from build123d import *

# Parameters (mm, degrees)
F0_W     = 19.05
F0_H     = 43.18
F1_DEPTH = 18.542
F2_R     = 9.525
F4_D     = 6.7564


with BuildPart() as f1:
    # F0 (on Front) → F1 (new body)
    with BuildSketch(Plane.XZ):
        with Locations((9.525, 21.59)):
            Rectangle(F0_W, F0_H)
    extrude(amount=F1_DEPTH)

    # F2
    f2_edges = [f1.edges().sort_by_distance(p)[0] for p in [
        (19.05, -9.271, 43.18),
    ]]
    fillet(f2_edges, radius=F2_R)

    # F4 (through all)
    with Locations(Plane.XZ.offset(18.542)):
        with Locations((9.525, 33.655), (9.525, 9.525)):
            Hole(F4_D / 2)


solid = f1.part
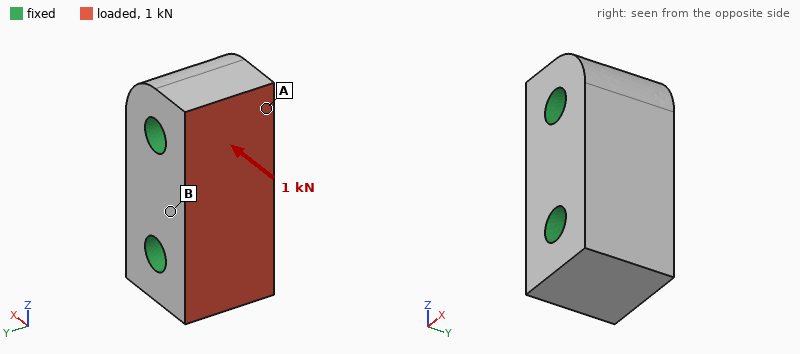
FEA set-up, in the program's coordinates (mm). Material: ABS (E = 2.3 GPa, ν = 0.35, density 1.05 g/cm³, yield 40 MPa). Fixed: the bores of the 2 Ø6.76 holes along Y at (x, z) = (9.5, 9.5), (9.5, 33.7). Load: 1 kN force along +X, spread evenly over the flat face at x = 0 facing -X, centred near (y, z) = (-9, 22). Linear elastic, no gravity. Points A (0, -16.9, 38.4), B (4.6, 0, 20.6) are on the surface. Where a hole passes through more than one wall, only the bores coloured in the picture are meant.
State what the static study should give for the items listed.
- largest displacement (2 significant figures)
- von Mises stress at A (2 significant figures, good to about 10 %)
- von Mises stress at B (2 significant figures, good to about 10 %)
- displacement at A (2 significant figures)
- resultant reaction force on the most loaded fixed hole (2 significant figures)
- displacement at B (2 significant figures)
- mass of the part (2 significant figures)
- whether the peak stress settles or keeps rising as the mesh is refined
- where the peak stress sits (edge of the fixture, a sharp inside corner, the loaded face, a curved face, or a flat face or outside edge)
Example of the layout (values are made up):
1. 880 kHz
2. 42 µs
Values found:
1. 10 µm
2. 1.5 MPa
3. 0.86 MPa
4. 7.2 µm
5. 500 N
6. 6.9 µm
7. 14 g
8. keeps rising
9. edge of the fixture
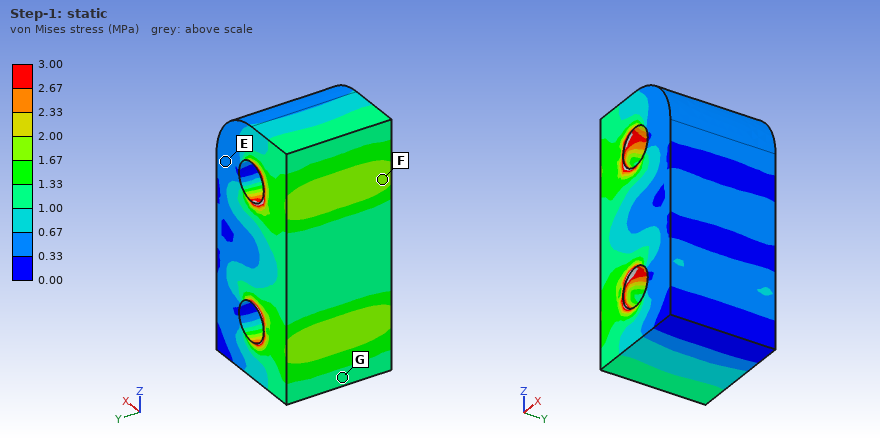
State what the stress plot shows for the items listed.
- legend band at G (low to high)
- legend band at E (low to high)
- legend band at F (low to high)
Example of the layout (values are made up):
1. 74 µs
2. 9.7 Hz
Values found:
1. 1.00 to 1.33 MPa
2. 0.33 to 0.67 MPa
3. 1.67 to 2.00 MPa
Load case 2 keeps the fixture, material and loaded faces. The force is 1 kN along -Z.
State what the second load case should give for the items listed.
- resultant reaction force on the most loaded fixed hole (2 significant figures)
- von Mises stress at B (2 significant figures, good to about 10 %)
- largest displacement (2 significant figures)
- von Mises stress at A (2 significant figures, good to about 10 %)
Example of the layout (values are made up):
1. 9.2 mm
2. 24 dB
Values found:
1. 560 N
2. 2.3 MPa
3. 29 µm
4. 2.7 MPa
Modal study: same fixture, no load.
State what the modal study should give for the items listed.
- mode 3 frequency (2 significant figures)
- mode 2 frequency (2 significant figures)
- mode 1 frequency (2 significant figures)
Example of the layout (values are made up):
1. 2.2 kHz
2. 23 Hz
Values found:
1. 18 kHz
2. 18 kHz
3. 17 kHz
